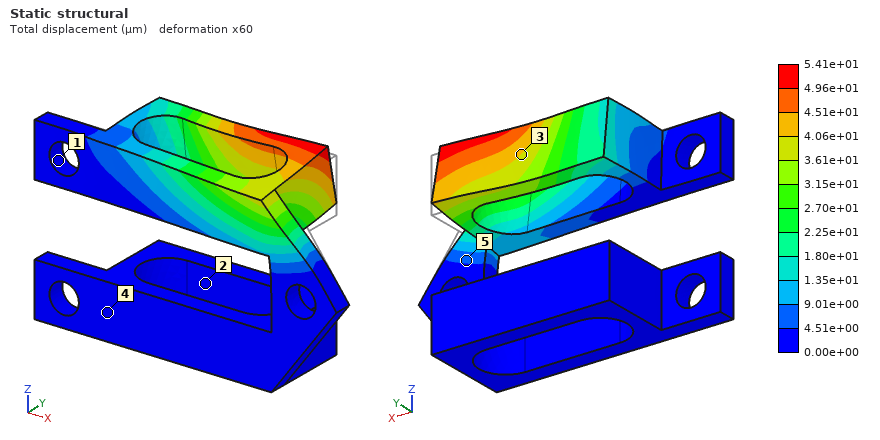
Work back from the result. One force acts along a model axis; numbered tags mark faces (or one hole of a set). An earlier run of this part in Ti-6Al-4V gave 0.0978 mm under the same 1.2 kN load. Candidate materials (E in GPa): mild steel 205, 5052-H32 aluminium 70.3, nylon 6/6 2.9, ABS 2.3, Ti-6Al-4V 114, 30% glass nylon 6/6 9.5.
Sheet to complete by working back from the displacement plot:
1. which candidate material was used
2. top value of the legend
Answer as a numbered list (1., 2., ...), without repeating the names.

1. mild steel
2. 5.41e+01 µm
